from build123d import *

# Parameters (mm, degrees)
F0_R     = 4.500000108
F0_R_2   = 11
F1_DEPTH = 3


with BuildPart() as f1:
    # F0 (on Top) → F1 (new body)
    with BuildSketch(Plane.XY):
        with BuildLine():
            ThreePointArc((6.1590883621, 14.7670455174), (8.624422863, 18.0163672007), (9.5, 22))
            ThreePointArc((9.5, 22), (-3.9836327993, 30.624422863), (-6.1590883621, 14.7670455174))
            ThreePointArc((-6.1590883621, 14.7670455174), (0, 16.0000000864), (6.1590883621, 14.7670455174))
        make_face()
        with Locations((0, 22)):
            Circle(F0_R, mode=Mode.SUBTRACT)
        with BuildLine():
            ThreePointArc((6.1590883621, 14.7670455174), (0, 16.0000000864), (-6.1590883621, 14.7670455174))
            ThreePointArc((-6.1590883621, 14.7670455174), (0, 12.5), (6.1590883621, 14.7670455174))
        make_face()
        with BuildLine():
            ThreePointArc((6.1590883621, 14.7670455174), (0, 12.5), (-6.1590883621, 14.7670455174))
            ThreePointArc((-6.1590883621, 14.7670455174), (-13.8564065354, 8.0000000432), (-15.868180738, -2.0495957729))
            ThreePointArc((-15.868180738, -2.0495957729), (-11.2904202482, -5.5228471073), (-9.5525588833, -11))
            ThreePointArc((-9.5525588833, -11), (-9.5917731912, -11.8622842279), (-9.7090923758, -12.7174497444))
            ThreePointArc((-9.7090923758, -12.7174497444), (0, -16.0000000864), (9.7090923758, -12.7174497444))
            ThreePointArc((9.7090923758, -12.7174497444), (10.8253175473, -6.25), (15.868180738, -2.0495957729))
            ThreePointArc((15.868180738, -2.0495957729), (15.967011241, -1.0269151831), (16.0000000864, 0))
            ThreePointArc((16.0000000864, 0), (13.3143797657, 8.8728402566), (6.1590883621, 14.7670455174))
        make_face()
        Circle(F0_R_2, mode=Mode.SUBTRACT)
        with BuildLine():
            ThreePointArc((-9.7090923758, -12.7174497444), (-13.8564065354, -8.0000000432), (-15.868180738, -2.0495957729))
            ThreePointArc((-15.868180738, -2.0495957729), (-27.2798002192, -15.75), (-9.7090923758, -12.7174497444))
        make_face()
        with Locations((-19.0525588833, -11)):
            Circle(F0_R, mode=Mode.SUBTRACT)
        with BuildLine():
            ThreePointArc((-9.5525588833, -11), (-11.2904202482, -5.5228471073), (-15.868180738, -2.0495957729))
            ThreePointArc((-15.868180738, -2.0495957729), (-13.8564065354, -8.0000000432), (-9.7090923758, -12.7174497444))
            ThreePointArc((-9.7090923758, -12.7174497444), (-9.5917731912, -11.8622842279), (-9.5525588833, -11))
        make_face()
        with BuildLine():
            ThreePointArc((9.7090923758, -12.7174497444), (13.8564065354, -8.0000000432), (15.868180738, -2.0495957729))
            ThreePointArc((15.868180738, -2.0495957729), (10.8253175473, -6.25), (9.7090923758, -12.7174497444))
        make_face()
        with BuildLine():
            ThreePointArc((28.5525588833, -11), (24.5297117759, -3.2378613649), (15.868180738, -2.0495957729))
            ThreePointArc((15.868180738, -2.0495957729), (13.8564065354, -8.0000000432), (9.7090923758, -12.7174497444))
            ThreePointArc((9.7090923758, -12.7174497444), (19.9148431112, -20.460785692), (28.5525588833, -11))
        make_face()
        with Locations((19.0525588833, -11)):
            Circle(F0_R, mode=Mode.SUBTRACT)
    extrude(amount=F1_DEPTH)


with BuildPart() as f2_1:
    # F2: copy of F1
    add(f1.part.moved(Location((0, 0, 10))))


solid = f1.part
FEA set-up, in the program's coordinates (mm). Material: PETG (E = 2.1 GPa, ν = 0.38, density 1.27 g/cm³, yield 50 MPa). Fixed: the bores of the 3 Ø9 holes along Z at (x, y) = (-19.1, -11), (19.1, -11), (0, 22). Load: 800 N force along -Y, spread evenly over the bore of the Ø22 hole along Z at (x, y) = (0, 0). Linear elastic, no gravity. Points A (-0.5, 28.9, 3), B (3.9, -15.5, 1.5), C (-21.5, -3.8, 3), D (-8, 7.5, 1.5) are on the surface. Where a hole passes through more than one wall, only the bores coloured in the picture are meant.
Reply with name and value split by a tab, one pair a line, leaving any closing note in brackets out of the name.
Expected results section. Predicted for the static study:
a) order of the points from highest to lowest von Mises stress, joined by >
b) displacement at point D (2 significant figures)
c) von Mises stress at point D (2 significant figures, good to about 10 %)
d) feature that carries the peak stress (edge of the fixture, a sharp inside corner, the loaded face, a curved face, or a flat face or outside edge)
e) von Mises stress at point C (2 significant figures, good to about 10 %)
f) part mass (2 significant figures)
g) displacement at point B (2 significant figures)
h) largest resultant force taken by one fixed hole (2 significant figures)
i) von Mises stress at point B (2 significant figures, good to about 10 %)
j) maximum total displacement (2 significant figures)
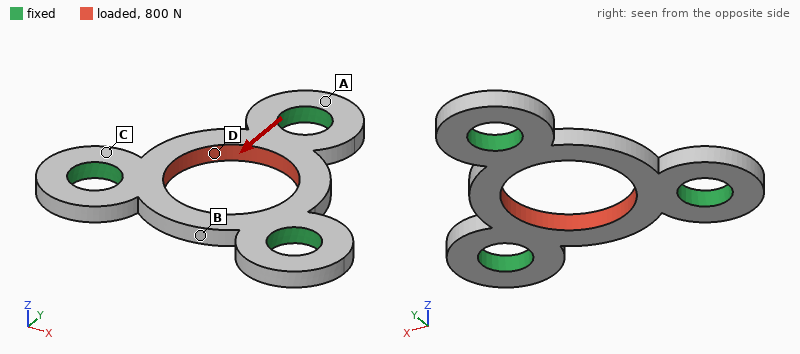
order of the points from highest to lowest von Mises stress, joined by >	B > D > C > A
displacement at point D	0.086 mm
von Mises stress at point D	7.3 MPa
feature that carries the peak stress	edge of the fixture
von Mises stress at point C	3.6 MPa
part mass	3.8 g
displacement at point B	0.15 mm
largest resultant force taken by one fixed hole	290 N
von Mises stress at point B	14 MPa
maximum total displacement	0.18 mm
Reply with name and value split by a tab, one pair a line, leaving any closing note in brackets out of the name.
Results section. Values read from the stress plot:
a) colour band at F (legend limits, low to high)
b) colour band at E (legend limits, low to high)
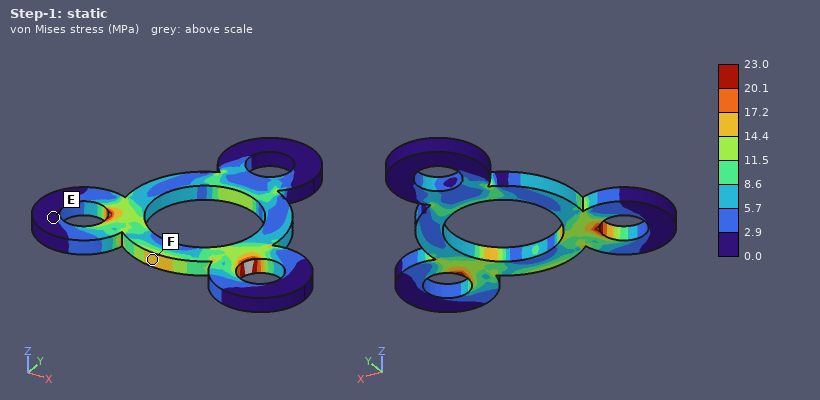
colour band at F	14.4 to 17.2 MPa
colour band at E	0.0 to 2.9 MPa
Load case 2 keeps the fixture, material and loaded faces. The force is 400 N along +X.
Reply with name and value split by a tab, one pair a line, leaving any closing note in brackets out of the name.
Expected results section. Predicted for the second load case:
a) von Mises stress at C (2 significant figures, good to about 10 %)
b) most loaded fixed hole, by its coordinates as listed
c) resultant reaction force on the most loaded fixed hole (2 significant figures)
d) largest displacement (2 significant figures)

von Mises stress at C	2.1 MPa
most loaded fixed hole, by its coordinates as listed	(0, 22)
resultant reaction force on the most loaded fixed hole	160 N
largest displacement	81 µm
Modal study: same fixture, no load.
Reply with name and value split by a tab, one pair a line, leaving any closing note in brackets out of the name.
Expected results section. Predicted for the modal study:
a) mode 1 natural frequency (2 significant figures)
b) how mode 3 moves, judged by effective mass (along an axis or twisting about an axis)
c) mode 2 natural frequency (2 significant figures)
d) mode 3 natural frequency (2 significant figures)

mode 1 natural frequency	4600 Hz
how mode 3 moves, judged by effective mass	along Z
mode 2 natural frequency	4600 Hz
mode 3 natural frequency	4800 Hz
